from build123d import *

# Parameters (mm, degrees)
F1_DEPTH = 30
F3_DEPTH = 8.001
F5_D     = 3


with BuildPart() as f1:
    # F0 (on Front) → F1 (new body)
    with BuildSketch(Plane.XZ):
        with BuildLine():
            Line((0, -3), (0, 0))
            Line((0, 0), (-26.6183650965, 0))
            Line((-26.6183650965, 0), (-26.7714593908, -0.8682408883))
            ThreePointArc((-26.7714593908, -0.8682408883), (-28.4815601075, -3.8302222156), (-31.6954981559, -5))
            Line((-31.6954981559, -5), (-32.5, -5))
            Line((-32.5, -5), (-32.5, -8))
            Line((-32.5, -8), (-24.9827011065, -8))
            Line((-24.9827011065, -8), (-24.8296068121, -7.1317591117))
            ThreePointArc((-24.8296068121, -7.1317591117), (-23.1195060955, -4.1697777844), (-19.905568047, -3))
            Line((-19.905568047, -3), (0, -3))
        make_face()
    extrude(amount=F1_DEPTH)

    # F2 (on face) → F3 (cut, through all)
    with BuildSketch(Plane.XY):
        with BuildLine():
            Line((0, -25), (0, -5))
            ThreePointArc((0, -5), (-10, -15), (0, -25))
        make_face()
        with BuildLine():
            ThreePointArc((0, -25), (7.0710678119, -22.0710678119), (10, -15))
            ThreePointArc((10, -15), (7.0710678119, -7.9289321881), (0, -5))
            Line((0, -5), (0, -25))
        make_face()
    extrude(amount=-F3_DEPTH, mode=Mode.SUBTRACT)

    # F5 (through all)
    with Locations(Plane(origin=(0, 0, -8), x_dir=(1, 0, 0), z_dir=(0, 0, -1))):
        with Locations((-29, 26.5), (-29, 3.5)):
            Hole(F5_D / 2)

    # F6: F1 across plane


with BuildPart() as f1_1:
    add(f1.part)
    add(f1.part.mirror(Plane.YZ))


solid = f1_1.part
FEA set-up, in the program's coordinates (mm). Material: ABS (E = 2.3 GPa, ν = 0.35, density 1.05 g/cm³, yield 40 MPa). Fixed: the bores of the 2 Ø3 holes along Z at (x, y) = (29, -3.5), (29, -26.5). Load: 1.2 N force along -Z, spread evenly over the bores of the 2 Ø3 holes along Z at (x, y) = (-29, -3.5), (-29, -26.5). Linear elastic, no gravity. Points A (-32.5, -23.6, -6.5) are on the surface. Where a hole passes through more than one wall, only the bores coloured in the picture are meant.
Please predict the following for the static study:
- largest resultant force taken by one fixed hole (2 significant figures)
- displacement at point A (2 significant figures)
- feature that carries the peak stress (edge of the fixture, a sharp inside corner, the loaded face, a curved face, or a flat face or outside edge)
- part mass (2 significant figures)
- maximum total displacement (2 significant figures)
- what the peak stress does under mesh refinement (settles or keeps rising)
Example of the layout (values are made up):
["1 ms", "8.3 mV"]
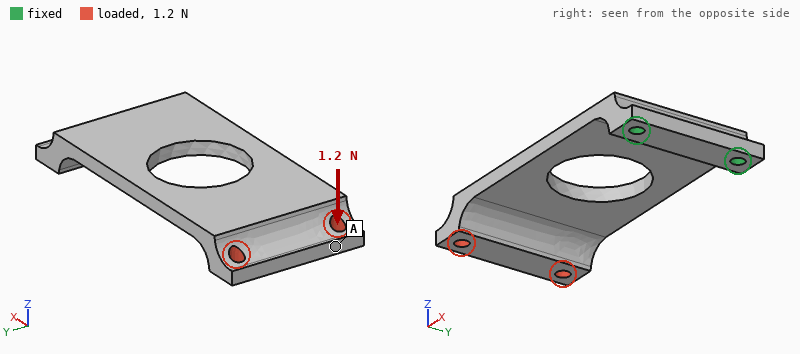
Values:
["0.95 N", "0.69 mm", "edge of the fixture", "6.3 g", "0.69 mm", "keeps rising"]
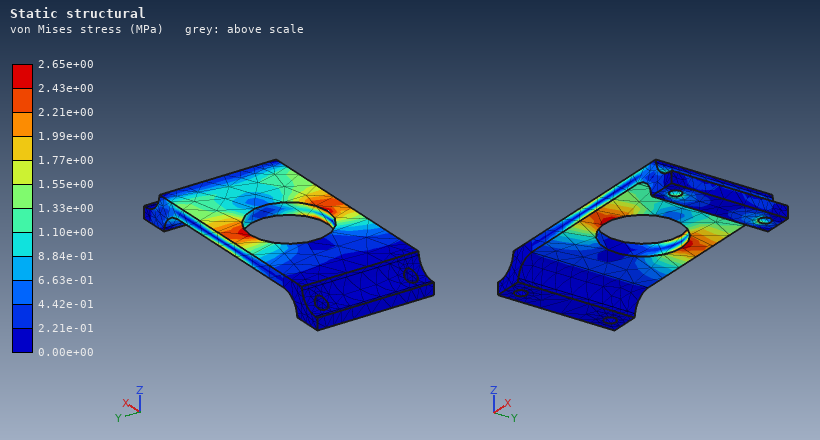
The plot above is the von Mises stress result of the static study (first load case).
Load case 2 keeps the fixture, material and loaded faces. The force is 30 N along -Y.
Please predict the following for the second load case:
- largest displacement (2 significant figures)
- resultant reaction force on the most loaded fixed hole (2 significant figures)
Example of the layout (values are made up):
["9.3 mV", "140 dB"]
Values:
["0.81 mm", "75 N"]
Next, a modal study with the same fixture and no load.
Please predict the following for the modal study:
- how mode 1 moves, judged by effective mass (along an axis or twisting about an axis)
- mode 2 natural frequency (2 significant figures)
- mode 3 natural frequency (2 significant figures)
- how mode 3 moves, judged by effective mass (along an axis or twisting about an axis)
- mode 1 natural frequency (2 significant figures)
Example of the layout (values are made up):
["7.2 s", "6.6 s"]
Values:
["along Z", "630 Hz", "1100 Hz", "along Y", "160 Hz"]
